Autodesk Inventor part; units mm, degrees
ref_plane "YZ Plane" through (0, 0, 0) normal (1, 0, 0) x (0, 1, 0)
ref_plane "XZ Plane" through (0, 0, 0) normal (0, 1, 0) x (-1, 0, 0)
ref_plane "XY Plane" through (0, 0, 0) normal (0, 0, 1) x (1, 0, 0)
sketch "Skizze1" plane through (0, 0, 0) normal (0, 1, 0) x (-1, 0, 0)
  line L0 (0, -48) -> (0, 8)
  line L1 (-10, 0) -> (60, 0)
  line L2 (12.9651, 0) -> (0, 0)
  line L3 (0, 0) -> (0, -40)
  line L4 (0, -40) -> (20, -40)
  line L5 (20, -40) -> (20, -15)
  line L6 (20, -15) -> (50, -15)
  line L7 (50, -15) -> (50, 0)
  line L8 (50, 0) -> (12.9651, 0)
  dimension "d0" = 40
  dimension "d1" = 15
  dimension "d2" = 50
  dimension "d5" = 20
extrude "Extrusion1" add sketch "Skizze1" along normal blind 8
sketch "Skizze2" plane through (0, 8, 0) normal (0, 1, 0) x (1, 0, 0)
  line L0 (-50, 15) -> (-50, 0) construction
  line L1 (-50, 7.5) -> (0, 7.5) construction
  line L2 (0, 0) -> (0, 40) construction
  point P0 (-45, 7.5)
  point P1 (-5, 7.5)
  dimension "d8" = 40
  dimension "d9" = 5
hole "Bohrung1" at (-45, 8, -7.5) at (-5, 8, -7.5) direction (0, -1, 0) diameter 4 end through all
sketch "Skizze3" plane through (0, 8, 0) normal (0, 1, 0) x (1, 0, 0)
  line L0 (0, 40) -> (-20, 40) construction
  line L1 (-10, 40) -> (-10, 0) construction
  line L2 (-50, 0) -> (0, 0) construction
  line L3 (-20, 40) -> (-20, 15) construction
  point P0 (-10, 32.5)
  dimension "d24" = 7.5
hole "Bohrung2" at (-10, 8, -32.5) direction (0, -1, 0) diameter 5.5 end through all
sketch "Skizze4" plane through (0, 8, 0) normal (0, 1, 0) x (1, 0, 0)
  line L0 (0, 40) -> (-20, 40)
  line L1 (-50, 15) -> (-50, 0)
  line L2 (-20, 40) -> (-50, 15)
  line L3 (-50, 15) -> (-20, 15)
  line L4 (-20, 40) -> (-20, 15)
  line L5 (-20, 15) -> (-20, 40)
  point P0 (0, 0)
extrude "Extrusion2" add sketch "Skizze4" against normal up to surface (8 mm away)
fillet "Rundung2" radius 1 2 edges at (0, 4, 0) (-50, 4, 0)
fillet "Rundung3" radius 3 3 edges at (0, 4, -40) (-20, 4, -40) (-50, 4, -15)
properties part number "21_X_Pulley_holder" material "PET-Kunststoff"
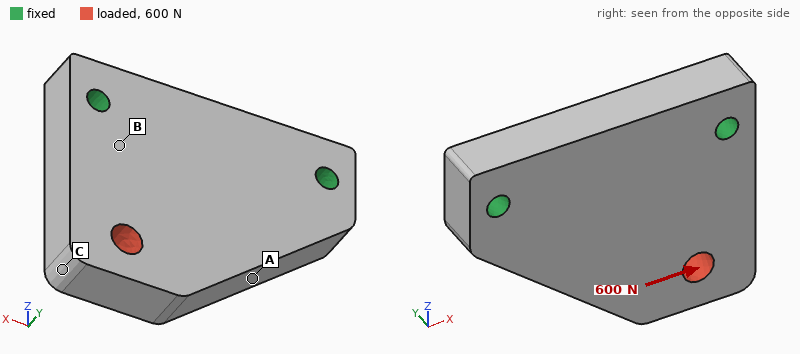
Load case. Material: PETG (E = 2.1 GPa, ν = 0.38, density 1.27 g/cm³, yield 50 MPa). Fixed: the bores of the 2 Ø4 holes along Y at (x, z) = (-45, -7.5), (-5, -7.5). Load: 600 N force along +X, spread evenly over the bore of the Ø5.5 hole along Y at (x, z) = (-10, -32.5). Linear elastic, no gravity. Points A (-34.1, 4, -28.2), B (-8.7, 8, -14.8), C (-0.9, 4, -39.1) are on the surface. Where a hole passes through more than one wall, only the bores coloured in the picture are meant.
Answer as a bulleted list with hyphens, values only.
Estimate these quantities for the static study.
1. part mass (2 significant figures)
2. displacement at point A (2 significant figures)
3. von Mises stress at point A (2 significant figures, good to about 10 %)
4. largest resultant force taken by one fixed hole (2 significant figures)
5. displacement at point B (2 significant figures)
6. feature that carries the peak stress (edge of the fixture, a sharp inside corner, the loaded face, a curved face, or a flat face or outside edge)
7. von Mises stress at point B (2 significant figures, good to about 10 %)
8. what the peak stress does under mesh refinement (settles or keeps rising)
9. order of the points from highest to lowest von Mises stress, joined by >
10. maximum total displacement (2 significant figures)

- 16 g
- 0.063 mm
- 5.7 MPa
- 500 N
- 0.024 mm
- edge of the fixture
- 3.6 MPa
- keeps rising
- A > B > C
- 0.14 mm
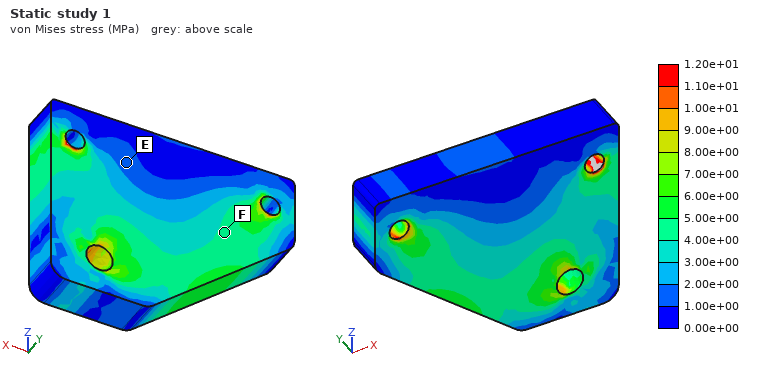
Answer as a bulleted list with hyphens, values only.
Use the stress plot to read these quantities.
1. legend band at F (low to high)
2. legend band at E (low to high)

- 4.00e+00 to 5.00e+00 MPa
- 1.00e+00 to 2.00e+00 MPa
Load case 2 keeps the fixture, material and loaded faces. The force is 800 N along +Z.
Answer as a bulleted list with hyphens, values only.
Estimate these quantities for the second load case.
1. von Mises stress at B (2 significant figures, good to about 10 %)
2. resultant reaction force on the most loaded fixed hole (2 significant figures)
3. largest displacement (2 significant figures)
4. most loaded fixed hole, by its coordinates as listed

- 6.2 MPa
- 700 N
- 0.10 mm
- (-5, -7.5)
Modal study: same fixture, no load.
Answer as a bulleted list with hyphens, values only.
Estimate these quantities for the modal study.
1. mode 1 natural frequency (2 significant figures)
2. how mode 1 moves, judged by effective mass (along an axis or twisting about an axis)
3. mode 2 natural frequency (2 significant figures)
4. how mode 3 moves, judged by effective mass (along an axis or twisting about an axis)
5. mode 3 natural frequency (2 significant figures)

- 1500 Hz
- along Y
- 3700 Hz
- along X
- 5400 Hz
